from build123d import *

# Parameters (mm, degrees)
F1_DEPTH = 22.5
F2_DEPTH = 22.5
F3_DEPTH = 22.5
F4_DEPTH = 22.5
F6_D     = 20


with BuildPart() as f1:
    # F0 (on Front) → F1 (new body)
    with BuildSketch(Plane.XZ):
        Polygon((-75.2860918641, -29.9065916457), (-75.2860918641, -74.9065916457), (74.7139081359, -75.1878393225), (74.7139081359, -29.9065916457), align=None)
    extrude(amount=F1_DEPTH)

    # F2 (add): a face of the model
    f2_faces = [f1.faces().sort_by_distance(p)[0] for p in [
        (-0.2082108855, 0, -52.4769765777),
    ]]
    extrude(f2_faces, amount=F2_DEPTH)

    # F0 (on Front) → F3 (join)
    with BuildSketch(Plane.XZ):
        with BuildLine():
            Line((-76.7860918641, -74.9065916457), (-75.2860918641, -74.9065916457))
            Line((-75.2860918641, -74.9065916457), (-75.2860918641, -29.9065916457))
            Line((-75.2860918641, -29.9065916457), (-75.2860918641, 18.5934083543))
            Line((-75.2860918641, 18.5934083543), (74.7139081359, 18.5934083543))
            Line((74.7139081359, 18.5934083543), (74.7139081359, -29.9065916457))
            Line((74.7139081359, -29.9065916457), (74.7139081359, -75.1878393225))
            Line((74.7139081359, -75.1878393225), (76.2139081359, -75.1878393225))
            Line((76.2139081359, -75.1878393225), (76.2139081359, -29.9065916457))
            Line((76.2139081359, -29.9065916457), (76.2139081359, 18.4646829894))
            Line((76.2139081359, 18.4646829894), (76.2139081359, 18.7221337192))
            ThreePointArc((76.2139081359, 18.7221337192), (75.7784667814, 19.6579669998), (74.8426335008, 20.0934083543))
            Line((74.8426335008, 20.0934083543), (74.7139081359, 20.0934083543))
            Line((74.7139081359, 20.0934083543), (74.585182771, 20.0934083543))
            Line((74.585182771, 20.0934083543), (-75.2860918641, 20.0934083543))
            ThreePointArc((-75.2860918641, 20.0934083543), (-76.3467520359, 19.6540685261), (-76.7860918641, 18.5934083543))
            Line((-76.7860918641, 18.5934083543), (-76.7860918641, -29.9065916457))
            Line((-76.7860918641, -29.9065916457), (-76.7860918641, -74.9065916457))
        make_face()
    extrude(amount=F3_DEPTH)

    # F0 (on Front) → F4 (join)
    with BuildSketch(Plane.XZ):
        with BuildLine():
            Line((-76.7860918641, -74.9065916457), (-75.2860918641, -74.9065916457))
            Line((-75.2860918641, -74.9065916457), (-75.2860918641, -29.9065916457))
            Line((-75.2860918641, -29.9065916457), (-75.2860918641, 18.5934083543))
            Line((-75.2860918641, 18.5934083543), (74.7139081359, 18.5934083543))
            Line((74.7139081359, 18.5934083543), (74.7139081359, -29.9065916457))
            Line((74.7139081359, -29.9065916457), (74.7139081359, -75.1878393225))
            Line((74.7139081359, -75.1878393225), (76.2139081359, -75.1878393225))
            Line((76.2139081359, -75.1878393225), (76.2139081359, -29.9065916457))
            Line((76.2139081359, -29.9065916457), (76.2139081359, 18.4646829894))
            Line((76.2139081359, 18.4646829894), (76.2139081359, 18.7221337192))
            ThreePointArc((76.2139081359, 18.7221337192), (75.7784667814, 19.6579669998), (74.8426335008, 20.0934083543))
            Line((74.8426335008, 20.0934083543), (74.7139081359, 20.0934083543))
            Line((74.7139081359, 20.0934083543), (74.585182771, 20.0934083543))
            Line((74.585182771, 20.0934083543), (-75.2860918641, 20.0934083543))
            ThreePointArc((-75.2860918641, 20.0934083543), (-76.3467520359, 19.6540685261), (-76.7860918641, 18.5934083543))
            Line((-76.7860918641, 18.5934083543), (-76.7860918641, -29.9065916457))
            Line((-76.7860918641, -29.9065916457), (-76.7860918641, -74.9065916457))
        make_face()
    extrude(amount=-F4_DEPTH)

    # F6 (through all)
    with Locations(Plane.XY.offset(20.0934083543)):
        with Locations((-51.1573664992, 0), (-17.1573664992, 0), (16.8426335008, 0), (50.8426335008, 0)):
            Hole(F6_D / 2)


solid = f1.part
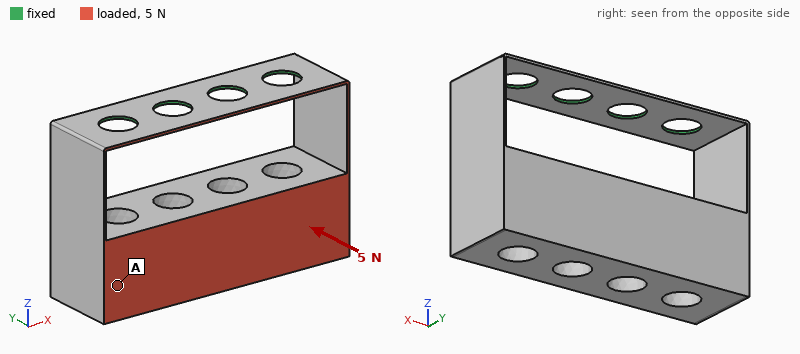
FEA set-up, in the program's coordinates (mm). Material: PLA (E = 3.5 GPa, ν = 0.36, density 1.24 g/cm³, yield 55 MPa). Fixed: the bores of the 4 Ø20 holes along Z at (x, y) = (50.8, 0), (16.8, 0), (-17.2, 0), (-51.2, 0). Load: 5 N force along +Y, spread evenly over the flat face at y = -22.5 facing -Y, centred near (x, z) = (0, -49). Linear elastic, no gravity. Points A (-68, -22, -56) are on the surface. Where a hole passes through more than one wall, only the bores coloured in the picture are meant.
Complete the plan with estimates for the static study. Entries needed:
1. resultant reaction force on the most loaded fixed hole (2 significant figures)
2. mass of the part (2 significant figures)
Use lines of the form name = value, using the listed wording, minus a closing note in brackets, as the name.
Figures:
resultant reaction force on the most loaded fixed hole = 3.0 N
mass of the part = 330 g
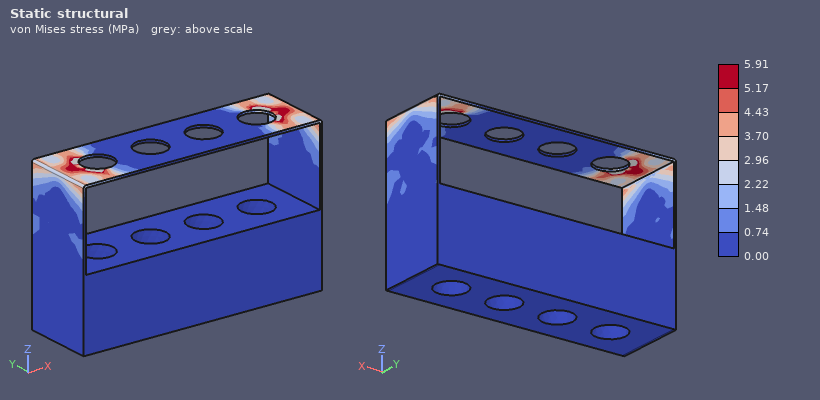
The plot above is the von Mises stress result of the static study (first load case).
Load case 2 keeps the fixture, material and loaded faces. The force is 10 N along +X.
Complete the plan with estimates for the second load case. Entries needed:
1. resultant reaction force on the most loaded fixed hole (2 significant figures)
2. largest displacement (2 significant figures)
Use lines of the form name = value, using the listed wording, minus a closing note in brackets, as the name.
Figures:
resultant reaction force on the most loaded fixed hole = 5.9 N
largest displacement = 2.1 mm
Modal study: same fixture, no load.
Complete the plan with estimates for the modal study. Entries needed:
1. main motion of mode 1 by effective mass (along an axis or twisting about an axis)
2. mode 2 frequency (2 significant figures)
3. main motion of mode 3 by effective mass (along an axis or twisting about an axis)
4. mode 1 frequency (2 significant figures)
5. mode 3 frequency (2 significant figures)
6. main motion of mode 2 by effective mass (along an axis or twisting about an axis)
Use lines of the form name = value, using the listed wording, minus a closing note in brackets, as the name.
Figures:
main motion of mode 1 by effective mass = along Y
mode 2 frequency = 20 Hz
main motion of mode 3 by effective mass = along Z
mode 1 frequency = 15 Hz
mode 3 frequency = 88 Hz
main motion of mode 2 by effective mass = along X
